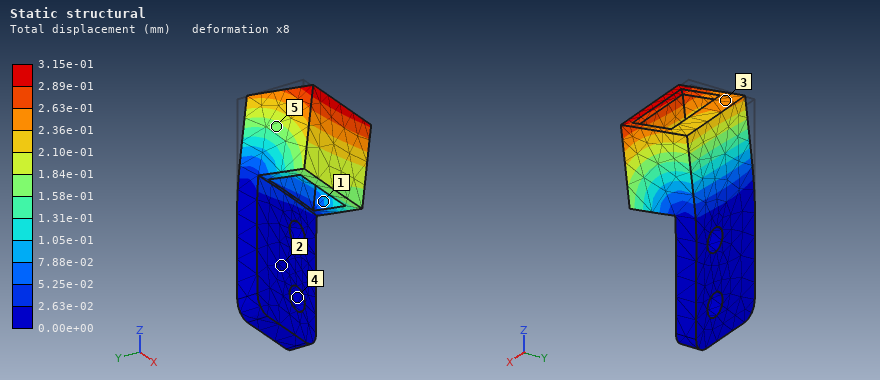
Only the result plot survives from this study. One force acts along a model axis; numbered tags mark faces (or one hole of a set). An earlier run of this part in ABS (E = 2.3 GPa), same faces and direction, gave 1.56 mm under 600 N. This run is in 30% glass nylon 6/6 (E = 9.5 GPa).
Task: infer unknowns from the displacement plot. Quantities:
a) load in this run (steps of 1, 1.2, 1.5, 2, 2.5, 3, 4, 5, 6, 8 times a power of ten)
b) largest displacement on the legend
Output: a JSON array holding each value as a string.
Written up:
["500 N", "3.15e-01 mm"]
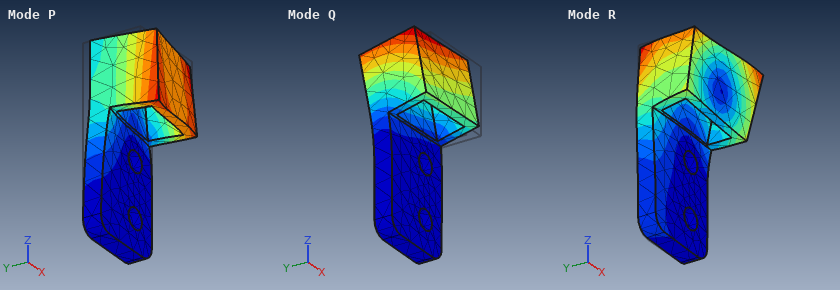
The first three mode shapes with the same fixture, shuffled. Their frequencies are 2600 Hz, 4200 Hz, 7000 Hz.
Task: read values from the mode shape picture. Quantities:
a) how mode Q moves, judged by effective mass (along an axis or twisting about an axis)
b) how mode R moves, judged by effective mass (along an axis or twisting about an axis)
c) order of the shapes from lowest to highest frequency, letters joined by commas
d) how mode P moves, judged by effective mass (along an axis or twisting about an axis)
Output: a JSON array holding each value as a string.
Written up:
["along Y", "along X", "Q, P, R", "along X"]
